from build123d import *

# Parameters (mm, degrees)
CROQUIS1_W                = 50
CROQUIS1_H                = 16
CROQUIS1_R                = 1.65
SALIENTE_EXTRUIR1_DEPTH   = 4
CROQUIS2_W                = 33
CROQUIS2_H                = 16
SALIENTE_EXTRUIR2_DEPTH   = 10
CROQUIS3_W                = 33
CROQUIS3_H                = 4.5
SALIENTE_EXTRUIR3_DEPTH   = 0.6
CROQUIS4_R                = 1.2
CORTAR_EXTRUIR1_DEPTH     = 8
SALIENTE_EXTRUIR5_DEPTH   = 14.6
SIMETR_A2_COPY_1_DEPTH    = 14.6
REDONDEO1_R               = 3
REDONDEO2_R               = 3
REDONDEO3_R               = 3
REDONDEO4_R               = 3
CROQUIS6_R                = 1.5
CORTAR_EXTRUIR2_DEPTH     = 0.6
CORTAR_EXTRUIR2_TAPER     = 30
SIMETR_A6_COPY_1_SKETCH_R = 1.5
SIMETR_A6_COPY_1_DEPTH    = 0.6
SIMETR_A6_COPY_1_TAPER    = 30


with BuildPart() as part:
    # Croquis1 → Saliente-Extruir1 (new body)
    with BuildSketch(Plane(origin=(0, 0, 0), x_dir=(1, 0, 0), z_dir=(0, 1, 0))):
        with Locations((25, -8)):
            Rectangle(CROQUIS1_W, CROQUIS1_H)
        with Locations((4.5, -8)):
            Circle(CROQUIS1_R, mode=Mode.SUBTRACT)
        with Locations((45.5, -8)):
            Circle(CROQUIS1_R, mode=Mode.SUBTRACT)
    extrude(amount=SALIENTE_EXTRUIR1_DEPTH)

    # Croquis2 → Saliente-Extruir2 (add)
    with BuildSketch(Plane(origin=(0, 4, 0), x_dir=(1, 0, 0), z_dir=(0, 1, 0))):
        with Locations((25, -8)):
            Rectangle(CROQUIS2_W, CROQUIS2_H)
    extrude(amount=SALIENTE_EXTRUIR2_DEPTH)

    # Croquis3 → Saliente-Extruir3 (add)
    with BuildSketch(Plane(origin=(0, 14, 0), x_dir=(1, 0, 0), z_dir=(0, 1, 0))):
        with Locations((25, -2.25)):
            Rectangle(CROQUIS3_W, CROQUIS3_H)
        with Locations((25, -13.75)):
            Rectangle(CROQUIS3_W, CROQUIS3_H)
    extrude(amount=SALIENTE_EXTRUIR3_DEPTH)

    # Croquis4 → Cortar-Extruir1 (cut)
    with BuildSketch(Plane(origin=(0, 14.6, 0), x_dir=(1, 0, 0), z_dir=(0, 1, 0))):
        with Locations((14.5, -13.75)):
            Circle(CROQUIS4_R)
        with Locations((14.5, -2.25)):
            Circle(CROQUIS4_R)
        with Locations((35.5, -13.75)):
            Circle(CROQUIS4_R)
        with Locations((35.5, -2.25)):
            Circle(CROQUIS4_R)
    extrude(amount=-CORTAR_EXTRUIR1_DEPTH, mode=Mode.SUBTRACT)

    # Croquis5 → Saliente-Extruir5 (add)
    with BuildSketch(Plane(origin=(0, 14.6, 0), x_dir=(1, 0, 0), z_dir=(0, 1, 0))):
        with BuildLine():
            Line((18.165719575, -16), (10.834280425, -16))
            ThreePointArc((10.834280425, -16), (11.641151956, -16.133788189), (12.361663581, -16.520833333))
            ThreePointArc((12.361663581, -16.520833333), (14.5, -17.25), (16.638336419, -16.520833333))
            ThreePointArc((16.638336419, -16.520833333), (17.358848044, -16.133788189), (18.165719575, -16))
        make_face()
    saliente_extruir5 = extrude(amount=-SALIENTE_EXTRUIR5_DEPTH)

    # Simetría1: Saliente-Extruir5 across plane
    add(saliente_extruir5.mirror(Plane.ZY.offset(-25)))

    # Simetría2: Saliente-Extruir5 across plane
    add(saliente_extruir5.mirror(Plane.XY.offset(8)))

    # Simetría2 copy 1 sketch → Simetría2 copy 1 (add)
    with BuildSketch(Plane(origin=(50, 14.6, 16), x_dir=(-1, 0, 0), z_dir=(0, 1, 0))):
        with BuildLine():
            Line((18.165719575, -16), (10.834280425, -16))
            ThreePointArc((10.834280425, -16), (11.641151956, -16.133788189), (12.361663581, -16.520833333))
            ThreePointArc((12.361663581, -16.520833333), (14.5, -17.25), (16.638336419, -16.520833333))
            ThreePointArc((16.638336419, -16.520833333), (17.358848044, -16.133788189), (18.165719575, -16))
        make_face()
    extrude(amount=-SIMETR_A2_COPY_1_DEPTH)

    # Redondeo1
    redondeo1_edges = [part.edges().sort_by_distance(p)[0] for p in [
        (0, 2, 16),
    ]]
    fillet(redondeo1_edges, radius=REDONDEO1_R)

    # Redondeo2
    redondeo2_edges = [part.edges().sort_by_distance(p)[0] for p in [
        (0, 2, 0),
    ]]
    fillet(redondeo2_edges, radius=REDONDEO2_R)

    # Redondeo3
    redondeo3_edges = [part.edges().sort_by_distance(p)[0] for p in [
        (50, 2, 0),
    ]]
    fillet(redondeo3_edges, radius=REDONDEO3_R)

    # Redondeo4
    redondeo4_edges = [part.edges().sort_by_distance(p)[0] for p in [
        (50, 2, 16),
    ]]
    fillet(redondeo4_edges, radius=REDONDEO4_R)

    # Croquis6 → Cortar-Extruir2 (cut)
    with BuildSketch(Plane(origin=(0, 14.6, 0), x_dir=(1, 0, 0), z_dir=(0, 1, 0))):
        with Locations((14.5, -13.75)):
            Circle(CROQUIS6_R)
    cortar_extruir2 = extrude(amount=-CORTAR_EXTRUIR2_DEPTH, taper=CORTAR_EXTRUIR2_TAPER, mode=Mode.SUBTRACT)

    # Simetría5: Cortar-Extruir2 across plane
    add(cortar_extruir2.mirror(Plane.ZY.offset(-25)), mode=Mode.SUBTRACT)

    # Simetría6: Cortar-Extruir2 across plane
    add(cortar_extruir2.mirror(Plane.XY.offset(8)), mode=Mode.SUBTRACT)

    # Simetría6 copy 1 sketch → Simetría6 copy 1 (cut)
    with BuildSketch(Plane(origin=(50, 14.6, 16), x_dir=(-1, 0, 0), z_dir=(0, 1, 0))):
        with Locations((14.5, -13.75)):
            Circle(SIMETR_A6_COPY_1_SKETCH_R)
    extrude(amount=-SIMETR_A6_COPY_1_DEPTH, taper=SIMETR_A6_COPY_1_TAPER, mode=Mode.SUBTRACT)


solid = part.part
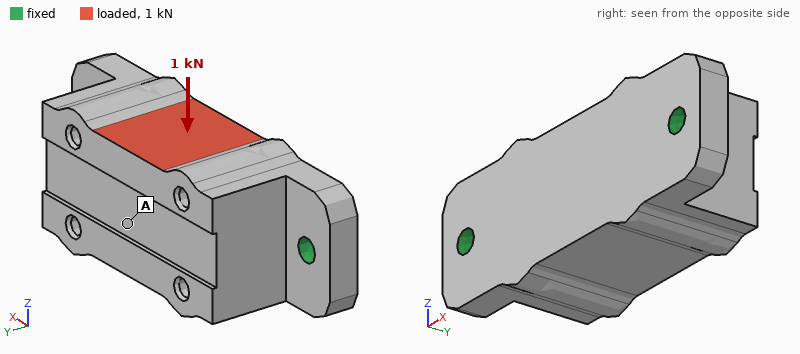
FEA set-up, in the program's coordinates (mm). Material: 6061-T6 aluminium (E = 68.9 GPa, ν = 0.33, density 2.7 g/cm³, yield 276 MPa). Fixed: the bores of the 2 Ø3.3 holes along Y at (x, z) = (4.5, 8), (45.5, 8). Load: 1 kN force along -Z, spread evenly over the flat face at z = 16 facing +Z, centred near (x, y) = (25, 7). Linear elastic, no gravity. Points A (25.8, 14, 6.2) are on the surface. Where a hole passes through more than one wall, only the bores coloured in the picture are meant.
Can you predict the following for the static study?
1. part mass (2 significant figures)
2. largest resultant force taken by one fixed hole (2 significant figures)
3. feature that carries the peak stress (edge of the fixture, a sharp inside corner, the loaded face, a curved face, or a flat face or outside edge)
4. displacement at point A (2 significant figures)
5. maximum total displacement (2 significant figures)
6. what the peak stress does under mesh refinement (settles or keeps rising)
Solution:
23 g
500 N
edge of the fixture
26 µm
31 µm
keeps rising
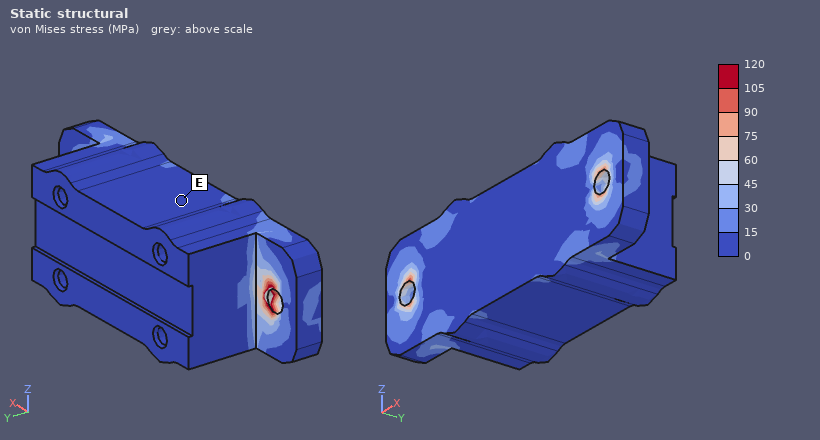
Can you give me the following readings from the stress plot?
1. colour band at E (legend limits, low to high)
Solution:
0 to 15 MPa
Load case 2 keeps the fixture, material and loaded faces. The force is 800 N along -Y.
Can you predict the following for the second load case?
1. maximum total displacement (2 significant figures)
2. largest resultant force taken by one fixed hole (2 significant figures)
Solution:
35 µm
500 N
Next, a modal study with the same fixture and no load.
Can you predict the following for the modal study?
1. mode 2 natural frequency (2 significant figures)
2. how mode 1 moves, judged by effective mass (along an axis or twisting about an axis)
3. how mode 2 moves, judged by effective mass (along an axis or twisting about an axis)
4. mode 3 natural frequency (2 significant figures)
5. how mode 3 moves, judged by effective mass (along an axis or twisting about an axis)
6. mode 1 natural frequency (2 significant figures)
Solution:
15 kHz
along Z
along Y
21 kHz
along Z
7300 Hz
